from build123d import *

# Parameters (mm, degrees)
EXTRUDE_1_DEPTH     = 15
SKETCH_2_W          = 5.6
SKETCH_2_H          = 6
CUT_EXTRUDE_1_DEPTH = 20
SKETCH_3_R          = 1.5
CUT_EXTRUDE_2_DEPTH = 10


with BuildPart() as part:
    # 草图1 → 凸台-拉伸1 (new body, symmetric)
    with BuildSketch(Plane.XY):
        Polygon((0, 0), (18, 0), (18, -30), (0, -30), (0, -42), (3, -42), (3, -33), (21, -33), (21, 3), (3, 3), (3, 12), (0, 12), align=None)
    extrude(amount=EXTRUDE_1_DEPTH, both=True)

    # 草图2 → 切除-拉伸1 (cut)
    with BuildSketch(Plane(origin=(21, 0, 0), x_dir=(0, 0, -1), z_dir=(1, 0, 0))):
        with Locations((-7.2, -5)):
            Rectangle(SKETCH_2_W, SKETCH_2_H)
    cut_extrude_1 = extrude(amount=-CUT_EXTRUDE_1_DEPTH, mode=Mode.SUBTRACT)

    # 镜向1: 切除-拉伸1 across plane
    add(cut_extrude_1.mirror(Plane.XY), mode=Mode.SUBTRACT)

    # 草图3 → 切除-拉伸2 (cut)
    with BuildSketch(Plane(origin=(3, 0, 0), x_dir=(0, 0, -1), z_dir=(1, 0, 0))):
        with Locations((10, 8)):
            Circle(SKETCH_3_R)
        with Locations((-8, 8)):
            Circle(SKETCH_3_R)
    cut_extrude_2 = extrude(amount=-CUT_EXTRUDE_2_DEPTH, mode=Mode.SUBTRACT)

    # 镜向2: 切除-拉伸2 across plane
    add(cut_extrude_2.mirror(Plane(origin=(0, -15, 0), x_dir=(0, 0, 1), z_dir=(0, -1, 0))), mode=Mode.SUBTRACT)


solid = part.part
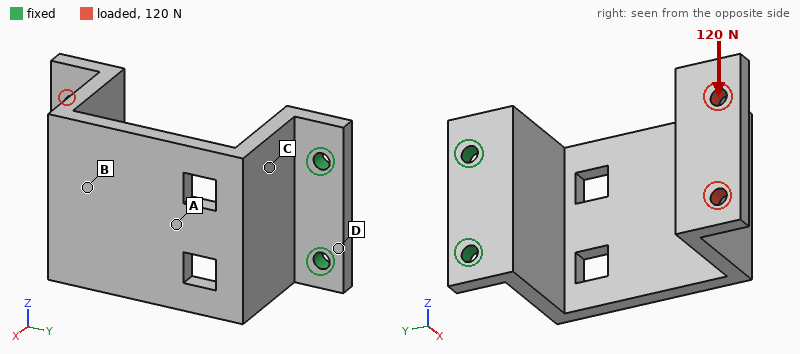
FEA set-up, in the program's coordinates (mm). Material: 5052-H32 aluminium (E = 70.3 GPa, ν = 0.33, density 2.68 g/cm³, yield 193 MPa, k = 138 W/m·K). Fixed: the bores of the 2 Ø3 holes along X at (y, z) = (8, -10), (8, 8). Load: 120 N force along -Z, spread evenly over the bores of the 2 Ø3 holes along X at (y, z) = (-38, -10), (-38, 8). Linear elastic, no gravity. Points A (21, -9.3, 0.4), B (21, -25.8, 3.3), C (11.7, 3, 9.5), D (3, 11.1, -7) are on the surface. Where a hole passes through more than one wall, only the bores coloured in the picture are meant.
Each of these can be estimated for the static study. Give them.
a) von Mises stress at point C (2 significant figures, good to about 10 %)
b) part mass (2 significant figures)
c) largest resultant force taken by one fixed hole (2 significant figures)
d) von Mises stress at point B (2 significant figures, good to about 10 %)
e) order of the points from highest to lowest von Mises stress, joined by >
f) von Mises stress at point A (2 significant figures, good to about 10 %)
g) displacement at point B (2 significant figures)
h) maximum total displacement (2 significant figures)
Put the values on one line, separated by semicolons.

69 MPa; 21 g; 280 N; 28 MPa; C > A > B > D; 52 MPa; 0.22 mm; 0.65 mm
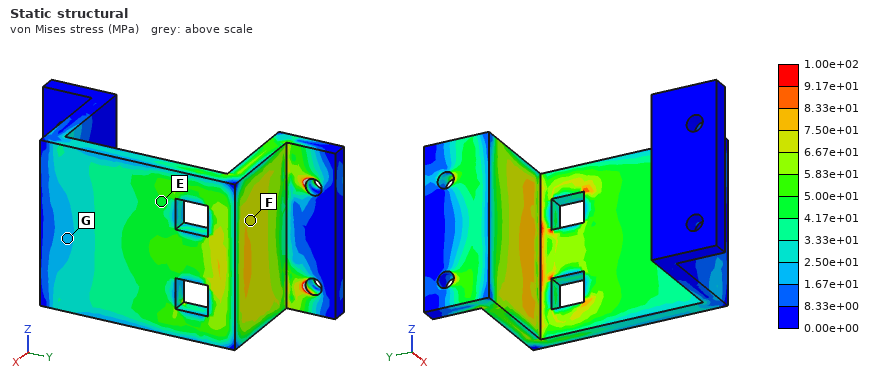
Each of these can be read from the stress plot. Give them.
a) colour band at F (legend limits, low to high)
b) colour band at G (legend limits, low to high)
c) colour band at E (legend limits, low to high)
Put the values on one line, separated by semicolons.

6.67e+01 to 7.50e+01 MPa; 1.67e+01 to 2.50e+01 MPa; 4.17e+01 to 5.00e+01 MPa
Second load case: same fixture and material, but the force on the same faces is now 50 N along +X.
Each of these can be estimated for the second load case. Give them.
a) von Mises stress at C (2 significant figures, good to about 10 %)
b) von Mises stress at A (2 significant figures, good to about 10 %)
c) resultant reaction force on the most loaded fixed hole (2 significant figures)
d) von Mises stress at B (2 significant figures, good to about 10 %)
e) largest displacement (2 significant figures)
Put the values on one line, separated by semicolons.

39 MPa; 38 MPa; 30 N; 13 MPa; 0.78 mm
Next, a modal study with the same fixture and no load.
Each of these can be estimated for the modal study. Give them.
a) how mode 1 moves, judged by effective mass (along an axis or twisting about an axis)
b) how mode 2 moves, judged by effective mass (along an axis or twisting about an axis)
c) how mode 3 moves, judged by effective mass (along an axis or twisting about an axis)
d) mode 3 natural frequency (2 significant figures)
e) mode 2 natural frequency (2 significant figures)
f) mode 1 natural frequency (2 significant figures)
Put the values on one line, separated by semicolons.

along X; along Z; along Y; 1600 Hz; 970 Hz; 520 Hz
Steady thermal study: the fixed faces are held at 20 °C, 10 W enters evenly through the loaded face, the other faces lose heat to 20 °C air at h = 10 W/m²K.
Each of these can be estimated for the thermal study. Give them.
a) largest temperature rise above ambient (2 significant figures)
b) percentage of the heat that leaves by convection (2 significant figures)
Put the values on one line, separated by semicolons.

62 K; 18 %
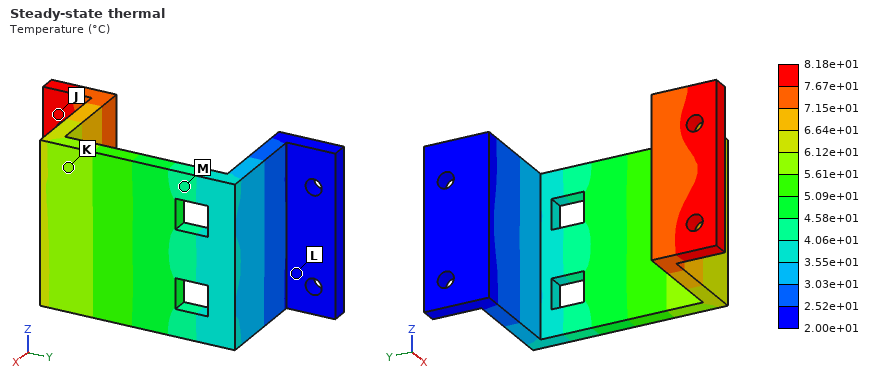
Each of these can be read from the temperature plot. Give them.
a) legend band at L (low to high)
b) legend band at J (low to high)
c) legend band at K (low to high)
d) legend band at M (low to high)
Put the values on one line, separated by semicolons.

2.00e+01 to 2.52e+01 °C; 7.67e+01 to 8.18e+01 °C; 5.61e+01 to 6.12e+01 °C; 4.06e+01 to 4.58e+01 °C
